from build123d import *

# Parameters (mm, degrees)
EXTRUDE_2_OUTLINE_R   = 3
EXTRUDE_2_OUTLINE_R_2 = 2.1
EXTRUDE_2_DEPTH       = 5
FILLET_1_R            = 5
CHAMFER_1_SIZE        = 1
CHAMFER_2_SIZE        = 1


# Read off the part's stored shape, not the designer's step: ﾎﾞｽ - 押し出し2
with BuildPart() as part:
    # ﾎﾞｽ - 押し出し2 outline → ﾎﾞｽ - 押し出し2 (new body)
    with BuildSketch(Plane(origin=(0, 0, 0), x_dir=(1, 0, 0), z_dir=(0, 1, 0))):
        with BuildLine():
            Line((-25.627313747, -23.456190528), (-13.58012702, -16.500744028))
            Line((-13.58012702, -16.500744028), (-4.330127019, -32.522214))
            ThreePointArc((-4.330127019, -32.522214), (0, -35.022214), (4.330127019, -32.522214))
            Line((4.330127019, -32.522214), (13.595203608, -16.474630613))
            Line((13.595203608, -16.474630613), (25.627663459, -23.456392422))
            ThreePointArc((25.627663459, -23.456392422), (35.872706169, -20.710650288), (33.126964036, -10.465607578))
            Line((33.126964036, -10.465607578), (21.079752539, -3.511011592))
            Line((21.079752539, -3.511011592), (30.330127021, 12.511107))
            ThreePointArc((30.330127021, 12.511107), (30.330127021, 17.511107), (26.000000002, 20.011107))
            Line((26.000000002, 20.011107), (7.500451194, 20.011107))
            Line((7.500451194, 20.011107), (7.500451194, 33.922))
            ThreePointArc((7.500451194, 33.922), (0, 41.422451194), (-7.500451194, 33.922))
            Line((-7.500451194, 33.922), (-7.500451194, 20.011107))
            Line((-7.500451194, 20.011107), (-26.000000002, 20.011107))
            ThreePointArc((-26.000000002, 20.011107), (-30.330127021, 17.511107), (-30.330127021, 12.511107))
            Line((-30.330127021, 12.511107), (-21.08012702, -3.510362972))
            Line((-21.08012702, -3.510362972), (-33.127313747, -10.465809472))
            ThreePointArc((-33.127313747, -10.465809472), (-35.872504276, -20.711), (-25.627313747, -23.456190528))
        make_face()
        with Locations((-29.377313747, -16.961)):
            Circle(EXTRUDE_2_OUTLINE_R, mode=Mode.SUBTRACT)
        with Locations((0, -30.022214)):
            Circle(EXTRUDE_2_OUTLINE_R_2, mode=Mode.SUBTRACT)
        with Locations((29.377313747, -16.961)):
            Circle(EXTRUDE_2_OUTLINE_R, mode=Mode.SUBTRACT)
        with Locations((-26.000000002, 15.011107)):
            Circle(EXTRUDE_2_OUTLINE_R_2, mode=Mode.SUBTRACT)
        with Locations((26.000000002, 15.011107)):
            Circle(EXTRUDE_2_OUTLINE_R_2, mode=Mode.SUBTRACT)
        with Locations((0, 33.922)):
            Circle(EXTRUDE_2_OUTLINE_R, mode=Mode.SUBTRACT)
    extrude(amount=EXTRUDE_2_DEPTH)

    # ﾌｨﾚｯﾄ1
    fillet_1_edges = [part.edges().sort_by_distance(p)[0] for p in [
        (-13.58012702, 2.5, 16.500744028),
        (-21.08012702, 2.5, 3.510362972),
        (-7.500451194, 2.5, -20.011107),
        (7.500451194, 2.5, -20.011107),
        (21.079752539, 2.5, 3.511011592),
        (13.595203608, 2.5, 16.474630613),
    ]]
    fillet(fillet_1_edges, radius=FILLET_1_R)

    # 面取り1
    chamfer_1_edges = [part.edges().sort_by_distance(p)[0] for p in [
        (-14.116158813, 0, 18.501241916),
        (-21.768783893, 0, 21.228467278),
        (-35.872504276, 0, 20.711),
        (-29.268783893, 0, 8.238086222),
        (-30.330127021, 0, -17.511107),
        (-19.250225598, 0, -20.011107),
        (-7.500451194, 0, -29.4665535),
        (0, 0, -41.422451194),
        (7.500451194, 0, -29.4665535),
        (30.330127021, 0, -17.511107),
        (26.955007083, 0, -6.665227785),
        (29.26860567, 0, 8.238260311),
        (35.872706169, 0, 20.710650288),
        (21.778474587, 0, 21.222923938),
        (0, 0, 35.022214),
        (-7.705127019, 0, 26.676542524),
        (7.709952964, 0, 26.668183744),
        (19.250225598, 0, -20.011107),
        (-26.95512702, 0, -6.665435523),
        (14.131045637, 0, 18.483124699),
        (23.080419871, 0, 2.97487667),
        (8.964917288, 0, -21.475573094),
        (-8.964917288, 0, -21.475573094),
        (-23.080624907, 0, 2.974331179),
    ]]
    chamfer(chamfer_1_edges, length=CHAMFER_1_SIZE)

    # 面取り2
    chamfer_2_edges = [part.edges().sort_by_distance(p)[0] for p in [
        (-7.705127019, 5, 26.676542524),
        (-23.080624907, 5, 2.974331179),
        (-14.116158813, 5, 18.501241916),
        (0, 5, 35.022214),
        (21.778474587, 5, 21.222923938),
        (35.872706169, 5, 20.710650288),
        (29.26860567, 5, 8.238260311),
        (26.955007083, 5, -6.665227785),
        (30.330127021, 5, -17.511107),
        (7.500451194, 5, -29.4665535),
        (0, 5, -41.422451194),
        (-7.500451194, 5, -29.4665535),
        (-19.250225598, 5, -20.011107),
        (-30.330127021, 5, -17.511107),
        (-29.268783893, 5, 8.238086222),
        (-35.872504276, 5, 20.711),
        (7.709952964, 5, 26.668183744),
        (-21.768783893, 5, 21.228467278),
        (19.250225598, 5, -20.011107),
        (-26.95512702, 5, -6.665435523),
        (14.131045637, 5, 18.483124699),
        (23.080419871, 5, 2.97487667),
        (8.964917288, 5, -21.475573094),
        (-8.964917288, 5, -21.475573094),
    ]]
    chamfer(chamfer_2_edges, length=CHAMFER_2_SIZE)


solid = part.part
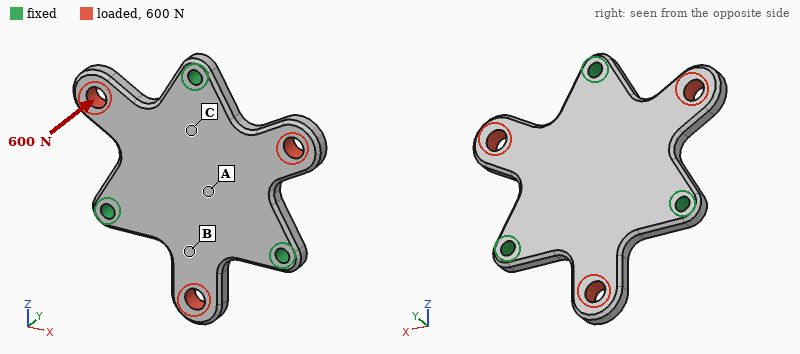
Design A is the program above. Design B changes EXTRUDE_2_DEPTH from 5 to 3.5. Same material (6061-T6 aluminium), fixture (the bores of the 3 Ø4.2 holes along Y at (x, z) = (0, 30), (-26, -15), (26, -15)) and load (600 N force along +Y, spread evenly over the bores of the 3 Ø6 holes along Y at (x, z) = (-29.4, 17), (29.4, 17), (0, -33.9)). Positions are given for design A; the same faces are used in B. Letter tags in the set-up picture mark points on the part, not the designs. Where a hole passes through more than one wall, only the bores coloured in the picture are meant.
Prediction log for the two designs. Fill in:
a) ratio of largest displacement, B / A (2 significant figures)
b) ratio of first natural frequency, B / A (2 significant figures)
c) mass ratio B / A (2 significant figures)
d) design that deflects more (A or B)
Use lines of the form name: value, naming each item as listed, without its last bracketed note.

ratio of largest displacement, B / A: 2.8
ratio of first natural frequency, B / A: 0.74
mass ratio B / A: 0.69
design that deflects more: B
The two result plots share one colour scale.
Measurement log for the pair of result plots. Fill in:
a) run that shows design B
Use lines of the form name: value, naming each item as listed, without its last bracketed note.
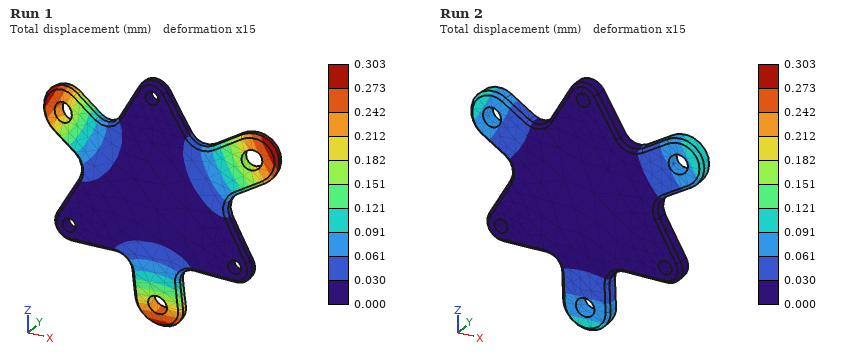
run that shows design B: Run 1
